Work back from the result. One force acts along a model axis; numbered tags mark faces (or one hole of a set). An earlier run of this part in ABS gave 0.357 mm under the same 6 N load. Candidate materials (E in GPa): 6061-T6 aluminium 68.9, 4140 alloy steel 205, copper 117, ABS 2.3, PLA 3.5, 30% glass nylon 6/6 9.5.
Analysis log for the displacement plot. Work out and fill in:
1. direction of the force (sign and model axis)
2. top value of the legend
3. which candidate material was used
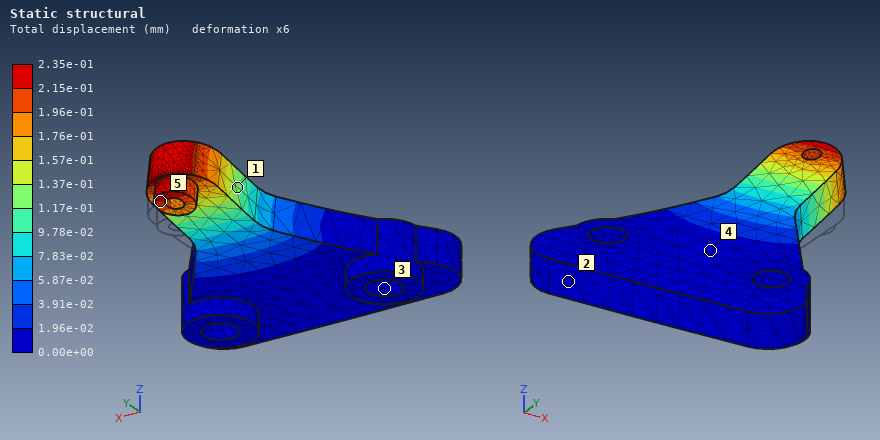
+Z
2.35e-01 mm
PLA
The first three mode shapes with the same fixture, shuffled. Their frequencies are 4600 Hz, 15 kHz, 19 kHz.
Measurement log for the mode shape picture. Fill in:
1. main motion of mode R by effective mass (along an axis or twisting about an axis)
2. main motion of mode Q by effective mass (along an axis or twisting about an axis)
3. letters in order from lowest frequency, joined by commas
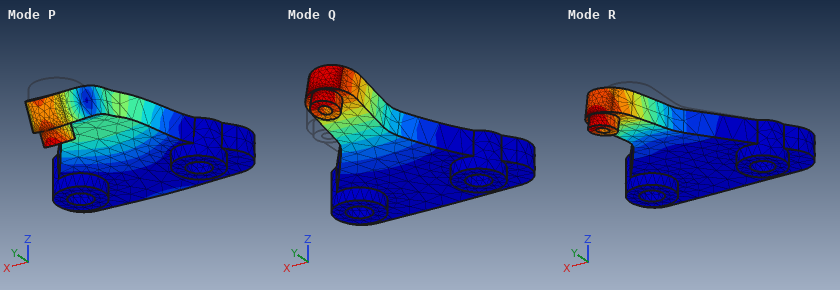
along X
along Z
Q, R, P
